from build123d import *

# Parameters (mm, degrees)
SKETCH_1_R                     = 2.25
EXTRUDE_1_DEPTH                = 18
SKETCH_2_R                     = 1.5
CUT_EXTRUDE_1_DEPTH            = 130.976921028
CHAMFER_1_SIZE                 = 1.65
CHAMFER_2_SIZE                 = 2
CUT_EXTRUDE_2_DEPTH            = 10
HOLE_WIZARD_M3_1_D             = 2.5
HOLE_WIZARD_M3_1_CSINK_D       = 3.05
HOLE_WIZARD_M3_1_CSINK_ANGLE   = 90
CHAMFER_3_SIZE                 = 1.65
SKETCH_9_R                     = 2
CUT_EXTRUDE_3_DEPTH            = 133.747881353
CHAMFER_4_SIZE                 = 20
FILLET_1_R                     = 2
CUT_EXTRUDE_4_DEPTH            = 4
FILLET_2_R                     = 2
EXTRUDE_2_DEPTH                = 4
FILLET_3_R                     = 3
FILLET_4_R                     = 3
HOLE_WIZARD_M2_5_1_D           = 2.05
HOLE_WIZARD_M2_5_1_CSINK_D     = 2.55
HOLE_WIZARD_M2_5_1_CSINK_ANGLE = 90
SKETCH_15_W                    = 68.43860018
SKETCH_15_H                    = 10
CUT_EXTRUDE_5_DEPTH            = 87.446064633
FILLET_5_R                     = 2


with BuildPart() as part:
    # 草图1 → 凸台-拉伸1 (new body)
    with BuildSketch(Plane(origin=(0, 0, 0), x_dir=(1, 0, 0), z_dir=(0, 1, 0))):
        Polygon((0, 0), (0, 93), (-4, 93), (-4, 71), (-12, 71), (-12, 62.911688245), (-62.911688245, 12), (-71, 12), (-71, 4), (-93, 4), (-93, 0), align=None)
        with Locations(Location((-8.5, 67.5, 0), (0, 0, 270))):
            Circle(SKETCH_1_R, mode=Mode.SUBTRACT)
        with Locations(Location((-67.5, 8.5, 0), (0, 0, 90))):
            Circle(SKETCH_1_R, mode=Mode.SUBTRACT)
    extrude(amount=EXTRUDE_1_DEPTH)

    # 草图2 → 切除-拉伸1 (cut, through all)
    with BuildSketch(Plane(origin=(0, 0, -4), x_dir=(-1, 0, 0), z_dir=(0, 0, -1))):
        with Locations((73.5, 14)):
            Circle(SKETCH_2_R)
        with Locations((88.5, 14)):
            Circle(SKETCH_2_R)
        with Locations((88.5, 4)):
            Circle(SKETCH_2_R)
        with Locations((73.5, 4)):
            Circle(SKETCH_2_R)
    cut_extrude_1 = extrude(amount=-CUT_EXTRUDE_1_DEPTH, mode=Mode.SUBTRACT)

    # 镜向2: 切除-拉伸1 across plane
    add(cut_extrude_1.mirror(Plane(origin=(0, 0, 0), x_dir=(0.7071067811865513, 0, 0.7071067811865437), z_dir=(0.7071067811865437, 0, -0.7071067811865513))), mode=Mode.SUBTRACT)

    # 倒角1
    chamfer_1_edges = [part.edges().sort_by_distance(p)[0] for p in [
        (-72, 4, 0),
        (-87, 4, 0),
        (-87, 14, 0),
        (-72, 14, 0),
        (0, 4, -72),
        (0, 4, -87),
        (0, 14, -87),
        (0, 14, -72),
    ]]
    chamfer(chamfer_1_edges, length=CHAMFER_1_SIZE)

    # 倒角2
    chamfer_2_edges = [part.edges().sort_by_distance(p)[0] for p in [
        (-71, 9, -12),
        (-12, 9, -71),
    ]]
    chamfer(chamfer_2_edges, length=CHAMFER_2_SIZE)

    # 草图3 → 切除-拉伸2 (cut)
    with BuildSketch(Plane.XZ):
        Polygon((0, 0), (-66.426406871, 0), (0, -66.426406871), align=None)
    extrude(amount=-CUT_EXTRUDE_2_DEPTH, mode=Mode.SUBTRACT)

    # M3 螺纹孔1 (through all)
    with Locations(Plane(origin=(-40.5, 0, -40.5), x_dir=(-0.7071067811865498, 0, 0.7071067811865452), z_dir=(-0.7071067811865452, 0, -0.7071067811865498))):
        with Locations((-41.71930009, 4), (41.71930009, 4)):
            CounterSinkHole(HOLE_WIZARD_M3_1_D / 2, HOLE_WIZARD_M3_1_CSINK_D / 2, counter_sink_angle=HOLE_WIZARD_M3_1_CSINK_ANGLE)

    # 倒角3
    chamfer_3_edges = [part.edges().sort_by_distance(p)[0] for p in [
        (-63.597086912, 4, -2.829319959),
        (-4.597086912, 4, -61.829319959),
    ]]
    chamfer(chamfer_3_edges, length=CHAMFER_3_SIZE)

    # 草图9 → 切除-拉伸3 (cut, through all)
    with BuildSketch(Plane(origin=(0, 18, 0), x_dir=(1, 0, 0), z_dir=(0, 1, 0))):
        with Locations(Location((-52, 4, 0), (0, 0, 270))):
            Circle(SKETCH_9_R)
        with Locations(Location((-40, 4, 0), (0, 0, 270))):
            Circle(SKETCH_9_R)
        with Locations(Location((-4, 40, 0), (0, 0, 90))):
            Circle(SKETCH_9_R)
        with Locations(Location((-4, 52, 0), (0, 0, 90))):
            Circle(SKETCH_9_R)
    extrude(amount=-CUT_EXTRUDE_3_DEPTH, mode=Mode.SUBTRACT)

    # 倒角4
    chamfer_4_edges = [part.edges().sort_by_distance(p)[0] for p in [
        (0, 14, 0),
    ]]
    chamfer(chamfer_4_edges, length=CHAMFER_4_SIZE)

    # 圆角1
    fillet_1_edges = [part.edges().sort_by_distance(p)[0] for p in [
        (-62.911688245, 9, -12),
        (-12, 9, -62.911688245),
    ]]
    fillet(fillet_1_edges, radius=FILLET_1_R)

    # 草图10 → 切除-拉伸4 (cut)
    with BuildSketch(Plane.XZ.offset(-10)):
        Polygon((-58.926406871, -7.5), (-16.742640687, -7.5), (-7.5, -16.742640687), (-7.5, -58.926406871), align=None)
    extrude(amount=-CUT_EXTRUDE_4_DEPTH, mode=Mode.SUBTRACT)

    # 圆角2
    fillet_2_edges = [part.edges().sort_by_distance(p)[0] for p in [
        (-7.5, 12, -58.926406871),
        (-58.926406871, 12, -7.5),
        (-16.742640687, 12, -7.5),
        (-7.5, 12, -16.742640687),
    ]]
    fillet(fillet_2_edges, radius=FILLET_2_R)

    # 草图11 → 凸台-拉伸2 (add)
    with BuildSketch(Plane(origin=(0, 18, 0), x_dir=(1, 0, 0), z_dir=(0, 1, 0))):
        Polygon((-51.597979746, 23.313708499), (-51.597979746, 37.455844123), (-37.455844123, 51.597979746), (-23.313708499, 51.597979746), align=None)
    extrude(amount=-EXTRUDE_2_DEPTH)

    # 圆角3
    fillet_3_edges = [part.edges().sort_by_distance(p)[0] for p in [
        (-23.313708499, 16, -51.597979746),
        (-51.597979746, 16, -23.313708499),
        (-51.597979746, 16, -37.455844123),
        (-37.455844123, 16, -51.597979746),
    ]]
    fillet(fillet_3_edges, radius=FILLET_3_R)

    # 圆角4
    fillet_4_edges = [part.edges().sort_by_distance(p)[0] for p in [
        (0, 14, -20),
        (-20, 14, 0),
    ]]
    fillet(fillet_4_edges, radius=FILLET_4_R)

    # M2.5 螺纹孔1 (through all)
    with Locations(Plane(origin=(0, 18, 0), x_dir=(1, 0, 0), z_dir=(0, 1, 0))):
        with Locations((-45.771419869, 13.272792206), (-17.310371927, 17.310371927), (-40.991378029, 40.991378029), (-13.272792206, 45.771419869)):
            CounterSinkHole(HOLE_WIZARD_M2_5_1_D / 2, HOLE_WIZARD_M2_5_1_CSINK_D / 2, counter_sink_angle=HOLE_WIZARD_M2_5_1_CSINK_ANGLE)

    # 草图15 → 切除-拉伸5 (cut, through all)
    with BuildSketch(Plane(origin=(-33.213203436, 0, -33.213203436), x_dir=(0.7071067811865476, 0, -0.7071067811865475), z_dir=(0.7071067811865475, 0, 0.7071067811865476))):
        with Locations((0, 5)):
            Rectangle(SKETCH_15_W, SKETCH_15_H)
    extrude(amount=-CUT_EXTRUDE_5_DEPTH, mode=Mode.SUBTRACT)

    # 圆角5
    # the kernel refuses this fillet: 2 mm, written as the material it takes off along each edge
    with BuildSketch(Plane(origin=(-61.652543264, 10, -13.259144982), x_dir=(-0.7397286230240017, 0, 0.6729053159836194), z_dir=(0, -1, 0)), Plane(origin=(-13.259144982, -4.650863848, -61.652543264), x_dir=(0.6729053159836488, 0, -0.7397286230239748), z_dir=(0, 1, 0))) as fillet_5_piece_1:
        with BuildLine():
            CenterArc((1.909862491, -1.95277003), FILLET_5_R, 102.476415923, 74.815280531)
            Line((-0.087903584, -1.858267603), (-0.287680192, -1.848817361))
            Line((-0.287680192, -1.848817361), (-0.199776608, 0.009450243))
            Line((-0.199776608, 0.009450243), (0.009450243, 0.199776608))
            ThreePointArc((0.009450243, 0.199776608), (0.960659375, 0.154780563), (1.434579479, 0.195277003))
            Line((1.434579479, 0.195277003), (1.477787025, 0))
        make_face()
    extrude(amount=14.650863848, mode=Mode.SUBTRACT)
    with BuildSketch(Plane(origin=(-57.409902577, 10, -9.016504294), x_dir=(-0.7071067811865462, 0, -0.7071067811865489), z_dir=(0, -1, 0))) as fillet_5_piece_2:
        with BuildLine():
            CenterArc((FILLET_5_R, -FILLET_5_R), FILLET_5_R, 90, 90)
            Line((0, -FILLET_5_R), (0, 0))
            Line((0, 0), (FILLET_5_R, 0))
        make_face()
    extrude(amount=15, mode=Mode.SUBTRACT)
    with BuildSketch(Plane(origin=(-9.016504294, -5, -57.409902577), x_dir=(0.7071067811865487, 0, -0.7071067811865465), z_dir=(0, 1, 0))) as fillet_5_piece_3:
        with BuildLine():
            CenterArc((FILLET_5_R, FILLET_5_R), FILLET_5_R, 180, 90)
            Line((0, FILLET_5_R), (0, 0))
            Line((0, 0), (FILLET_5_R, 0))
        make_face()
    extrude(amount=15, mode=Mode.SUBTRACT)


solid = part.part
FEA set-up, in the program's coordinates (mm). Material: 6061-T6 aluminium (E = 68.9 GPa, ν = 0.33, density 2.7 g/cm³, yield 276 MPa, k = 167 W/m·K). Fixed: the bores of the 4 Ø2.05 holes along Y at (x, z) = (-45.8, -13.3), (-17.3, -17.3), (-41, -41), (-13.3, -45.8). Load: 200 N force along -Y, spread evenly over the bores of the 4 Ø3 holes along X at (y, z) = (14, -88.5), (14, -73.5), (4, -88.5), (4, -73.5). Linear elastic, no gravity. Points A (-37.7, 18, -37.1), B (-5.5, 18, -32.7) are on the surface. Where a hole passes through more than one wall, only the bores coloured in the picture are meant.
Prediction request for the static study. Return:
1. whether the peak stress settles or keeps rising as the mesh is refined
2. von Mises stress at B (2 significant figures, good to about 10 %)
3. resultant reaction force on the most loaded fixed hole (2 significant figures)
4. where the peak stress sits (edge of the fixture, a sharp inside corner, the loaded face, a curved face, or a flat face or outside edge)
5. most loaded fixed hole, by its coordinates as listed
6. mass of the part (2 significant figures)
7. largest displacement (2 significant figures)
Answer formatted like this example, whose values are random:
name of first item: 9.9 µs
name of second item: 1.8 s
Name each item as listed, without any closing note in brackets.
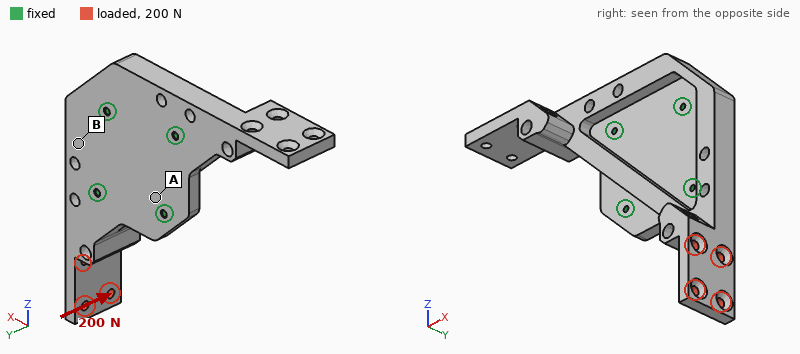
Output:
whether the peak stress settles or keeps rising as the mesh is refined: keeps rising
von Mises stress at B: 9.0 MPa
resultant reaction force on the most loaded fixed hole: 500 N
where the peak stress sits: edge of the fixture
most loaded fixed hole, by its coordinates as listed: (-13.3, -45.8)
mass of the part: 58 g
largest displacement: 0.20 mm
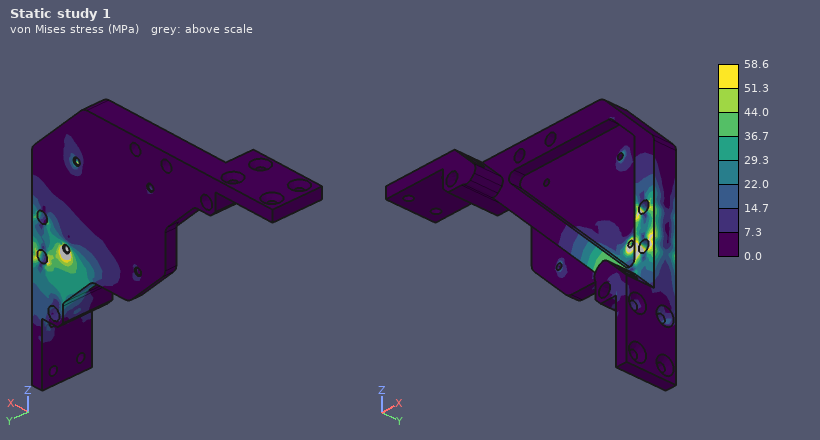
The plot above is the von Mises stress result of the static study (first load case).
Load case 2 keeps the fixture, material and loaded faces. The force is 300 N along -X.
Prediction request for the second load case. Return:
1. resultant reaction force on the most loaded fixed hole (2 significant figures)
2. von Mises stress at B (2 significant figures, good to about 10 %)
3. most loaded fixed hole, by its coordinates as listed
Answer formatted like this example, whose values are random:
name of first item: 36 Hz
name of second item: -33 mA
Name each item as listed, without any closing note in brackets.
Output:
resultant reaction force on the most loaded fixed hole: 310 N
von Mises stress at B: 6.3 MPa
most loaded fixed hole, by its coordinates as listed: (-13.3, -45.8)
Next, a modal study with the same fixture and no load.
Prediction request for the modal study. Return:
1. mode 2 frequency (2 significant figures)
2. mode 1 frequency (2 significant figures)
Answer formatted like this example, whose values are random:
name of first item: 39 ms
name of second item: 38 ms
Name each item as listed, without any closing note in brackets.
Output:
mode 2 frequency: 2500 Hz
mode 1 frequency: 2500 Hz
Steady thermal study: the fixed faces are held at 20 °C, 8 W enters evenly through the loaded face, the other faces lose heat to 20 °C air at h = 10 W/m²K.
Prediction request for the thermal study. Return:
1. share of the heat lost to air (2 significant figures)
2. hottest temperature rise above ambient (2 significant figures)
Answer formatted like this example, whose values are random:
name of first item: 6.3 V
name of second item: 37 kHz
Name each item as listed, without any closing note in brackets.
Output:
share of the heat lost to air: 5.1 %
hottest temperature rise above ambient: 23 K
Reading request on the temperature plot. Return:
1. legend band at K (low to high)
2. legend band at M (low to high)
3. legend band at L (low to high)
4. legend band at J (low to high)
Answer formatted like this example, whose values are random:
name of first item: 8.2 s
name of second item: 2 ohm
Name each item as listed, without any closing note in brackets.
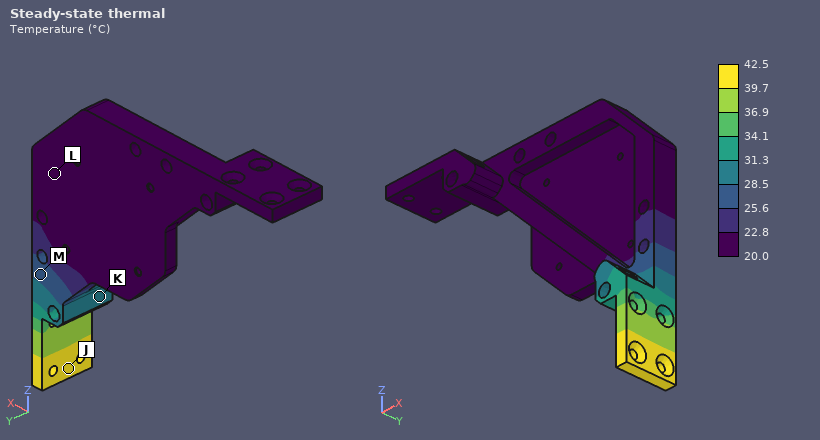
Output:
legend band at K: 28.5 to 31.3 °C
legend band at M: 25.6 to 28.5 °C
legend band at L: 20.0 to 22.8 °C
legend band at J: 39.7 to 42.5 °C
